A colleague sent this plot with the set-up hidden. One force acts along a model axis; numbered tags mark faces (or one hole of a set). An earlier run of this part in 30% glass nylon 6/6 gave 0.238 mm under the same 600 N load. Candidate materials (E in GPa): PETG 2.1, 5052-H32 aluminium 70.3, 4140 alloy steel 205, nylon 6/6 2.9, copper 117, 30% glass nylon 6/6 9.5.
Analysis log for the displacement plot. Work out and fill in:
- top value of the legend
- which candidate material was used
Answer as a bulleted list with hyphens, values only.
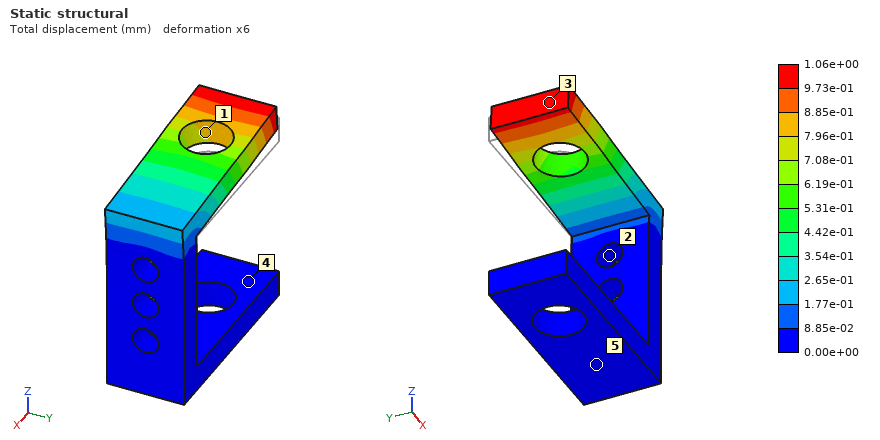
- 1.06e+00 mm
- PETG
